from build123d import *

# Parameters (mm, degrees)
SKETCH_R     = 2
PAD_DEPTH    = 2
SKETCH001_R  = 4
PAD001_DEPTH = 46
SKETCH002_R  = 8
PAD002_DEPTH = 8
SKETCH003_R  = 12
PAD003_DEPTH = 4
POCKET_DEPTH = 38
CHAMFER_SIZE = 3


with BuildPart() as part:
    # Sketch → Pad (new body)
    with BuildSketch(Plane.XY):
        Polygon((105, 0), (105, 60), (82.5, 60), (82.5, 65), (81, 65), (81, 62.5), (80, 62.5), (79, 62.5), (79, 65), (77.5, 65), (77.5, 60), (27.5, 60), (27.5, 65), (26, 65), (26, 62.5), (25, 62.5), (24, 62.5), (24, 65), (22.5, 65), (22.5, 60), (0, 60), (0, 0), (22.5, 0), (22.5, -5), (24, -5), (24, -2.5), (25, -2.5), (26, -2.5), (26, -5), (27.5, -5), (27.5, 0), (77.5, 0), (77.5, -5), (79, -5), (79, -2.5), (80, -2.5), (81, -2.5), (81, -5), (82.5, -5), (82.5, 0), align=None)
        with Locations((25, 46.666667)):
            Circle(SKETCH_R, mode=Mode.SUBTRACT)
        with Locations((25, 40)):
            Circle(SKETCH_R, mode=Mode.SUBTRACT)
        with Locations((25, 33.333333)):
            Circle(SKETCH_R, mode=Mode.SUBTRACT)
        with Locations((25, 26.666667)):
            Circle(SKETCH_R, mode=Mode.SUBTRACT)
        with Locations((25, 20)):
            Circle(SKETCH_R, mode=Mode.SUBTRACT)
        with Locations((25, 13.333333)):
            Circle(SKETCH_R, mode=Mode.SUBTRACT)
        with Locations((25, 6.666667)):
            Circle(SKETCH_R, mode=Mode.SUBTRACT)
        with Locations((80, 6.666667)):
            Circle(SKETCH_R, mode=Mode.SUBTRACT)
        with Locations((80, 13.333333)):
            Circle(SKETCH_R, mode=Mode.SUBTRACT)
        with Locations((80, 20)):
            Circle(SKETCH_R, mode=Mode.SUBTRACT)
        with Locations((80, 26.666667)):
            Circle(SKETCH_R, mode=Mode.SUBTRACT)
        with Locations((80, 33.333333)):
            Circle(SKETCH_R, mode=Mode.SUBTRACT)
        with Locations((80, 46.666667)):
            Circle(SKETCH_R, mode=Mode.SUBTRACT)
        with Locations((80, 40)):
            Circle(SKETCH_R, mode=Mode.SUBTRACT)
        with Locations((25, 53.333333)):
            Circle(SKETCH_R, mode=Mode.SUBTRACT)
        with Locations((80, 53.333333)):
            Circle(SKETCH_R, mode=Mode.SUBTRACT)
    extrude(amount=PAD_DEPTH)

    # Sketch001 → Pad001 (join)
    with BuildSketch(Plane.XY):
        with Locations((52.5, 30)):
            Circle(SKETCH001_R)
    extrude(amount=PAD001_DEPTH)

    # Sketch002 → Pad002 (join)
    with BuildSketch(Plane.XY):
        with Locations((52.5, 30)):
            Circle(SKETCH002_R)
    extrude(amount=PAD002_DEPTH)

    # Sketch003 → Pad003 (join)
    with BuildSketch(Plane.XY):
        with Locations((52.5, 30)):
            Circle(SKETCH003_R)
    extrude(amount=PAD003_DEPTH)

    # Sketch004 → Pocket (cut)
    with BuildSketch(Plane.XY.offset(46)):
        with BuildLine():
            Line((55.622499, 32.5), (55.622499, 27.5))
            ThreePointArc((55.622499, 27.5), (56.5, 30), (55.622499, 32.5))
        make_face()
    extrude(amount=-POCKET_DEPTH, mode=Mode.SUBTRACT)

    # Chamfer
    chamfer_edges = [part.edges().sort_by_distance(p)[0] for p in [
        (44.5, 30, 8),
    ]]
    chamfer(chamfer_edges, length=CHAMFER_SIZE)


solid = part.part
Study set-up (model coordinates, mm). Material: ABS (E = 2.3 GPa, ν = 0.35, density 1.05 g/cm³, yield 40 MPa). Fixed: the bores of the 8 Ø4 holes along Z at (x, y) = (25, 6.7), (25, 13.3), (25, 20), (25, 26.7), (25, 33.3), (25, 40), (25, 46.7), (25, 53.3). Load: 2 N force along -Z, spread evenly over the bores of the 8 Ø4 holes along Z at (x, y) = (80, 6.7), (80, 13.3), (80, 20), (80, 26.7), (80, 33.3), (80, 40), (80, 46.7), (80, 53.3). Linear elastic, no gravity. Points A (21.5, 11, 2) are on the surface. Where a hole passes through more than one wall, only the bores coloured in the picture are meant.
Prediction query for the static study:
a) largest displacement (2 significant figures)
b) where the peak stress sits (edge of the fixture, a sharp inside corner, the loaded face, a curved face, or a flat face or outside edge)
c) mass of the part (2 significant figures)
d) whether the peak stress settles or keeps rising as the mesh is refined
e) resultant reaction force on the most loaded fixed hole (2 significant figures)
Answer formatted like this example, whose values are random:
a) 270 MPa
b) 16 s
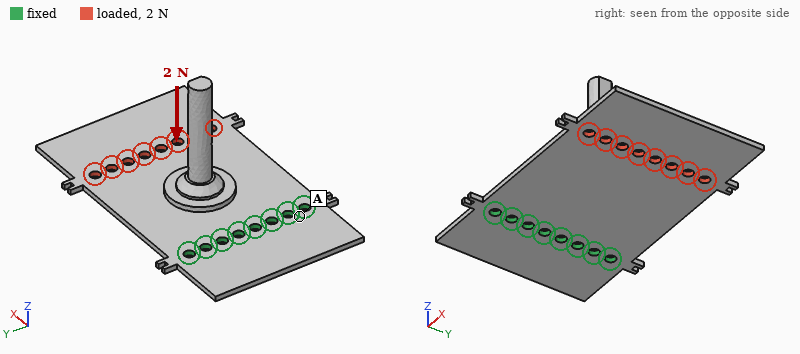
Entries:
a) 1.3 mm
b) edge of the fixture
c) 16 g
d) keeps rising
e) 1.0 N
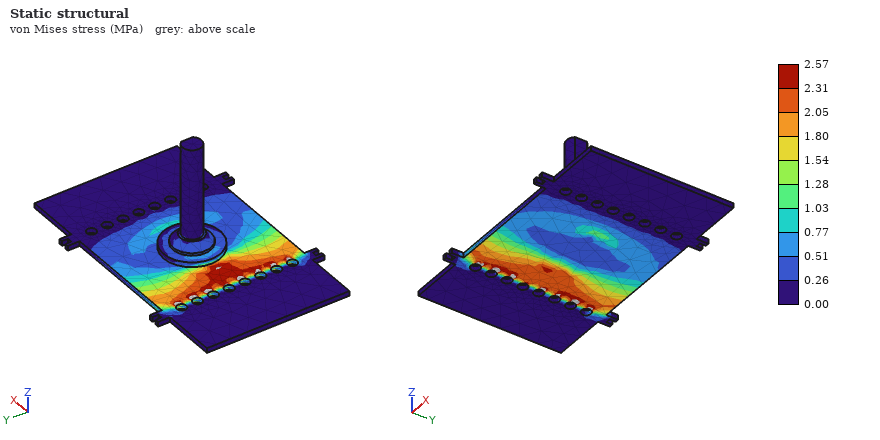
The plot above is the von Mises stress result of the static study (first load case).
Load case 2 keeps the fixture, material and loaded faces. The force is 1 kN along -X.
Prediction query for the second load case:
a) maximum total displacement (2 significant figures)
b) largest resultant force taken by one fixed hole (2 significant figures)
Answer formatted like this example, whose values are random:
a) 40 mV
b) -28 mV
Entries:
a) 0.95 mm
b) 170 N
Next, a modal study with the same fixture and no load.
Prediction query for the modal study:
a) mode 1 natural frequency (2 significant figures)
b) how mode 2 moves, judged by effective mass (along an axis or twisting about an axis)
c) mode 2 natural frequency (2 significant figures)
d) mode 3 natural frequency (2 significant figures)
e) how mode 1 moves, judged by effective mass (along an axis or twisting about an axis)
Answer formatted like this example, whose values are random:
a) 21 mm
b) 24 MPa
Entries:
a) 86 Hz
b) twisting about X
c) 280 Hz
d) 410 Hz
e) along Z
